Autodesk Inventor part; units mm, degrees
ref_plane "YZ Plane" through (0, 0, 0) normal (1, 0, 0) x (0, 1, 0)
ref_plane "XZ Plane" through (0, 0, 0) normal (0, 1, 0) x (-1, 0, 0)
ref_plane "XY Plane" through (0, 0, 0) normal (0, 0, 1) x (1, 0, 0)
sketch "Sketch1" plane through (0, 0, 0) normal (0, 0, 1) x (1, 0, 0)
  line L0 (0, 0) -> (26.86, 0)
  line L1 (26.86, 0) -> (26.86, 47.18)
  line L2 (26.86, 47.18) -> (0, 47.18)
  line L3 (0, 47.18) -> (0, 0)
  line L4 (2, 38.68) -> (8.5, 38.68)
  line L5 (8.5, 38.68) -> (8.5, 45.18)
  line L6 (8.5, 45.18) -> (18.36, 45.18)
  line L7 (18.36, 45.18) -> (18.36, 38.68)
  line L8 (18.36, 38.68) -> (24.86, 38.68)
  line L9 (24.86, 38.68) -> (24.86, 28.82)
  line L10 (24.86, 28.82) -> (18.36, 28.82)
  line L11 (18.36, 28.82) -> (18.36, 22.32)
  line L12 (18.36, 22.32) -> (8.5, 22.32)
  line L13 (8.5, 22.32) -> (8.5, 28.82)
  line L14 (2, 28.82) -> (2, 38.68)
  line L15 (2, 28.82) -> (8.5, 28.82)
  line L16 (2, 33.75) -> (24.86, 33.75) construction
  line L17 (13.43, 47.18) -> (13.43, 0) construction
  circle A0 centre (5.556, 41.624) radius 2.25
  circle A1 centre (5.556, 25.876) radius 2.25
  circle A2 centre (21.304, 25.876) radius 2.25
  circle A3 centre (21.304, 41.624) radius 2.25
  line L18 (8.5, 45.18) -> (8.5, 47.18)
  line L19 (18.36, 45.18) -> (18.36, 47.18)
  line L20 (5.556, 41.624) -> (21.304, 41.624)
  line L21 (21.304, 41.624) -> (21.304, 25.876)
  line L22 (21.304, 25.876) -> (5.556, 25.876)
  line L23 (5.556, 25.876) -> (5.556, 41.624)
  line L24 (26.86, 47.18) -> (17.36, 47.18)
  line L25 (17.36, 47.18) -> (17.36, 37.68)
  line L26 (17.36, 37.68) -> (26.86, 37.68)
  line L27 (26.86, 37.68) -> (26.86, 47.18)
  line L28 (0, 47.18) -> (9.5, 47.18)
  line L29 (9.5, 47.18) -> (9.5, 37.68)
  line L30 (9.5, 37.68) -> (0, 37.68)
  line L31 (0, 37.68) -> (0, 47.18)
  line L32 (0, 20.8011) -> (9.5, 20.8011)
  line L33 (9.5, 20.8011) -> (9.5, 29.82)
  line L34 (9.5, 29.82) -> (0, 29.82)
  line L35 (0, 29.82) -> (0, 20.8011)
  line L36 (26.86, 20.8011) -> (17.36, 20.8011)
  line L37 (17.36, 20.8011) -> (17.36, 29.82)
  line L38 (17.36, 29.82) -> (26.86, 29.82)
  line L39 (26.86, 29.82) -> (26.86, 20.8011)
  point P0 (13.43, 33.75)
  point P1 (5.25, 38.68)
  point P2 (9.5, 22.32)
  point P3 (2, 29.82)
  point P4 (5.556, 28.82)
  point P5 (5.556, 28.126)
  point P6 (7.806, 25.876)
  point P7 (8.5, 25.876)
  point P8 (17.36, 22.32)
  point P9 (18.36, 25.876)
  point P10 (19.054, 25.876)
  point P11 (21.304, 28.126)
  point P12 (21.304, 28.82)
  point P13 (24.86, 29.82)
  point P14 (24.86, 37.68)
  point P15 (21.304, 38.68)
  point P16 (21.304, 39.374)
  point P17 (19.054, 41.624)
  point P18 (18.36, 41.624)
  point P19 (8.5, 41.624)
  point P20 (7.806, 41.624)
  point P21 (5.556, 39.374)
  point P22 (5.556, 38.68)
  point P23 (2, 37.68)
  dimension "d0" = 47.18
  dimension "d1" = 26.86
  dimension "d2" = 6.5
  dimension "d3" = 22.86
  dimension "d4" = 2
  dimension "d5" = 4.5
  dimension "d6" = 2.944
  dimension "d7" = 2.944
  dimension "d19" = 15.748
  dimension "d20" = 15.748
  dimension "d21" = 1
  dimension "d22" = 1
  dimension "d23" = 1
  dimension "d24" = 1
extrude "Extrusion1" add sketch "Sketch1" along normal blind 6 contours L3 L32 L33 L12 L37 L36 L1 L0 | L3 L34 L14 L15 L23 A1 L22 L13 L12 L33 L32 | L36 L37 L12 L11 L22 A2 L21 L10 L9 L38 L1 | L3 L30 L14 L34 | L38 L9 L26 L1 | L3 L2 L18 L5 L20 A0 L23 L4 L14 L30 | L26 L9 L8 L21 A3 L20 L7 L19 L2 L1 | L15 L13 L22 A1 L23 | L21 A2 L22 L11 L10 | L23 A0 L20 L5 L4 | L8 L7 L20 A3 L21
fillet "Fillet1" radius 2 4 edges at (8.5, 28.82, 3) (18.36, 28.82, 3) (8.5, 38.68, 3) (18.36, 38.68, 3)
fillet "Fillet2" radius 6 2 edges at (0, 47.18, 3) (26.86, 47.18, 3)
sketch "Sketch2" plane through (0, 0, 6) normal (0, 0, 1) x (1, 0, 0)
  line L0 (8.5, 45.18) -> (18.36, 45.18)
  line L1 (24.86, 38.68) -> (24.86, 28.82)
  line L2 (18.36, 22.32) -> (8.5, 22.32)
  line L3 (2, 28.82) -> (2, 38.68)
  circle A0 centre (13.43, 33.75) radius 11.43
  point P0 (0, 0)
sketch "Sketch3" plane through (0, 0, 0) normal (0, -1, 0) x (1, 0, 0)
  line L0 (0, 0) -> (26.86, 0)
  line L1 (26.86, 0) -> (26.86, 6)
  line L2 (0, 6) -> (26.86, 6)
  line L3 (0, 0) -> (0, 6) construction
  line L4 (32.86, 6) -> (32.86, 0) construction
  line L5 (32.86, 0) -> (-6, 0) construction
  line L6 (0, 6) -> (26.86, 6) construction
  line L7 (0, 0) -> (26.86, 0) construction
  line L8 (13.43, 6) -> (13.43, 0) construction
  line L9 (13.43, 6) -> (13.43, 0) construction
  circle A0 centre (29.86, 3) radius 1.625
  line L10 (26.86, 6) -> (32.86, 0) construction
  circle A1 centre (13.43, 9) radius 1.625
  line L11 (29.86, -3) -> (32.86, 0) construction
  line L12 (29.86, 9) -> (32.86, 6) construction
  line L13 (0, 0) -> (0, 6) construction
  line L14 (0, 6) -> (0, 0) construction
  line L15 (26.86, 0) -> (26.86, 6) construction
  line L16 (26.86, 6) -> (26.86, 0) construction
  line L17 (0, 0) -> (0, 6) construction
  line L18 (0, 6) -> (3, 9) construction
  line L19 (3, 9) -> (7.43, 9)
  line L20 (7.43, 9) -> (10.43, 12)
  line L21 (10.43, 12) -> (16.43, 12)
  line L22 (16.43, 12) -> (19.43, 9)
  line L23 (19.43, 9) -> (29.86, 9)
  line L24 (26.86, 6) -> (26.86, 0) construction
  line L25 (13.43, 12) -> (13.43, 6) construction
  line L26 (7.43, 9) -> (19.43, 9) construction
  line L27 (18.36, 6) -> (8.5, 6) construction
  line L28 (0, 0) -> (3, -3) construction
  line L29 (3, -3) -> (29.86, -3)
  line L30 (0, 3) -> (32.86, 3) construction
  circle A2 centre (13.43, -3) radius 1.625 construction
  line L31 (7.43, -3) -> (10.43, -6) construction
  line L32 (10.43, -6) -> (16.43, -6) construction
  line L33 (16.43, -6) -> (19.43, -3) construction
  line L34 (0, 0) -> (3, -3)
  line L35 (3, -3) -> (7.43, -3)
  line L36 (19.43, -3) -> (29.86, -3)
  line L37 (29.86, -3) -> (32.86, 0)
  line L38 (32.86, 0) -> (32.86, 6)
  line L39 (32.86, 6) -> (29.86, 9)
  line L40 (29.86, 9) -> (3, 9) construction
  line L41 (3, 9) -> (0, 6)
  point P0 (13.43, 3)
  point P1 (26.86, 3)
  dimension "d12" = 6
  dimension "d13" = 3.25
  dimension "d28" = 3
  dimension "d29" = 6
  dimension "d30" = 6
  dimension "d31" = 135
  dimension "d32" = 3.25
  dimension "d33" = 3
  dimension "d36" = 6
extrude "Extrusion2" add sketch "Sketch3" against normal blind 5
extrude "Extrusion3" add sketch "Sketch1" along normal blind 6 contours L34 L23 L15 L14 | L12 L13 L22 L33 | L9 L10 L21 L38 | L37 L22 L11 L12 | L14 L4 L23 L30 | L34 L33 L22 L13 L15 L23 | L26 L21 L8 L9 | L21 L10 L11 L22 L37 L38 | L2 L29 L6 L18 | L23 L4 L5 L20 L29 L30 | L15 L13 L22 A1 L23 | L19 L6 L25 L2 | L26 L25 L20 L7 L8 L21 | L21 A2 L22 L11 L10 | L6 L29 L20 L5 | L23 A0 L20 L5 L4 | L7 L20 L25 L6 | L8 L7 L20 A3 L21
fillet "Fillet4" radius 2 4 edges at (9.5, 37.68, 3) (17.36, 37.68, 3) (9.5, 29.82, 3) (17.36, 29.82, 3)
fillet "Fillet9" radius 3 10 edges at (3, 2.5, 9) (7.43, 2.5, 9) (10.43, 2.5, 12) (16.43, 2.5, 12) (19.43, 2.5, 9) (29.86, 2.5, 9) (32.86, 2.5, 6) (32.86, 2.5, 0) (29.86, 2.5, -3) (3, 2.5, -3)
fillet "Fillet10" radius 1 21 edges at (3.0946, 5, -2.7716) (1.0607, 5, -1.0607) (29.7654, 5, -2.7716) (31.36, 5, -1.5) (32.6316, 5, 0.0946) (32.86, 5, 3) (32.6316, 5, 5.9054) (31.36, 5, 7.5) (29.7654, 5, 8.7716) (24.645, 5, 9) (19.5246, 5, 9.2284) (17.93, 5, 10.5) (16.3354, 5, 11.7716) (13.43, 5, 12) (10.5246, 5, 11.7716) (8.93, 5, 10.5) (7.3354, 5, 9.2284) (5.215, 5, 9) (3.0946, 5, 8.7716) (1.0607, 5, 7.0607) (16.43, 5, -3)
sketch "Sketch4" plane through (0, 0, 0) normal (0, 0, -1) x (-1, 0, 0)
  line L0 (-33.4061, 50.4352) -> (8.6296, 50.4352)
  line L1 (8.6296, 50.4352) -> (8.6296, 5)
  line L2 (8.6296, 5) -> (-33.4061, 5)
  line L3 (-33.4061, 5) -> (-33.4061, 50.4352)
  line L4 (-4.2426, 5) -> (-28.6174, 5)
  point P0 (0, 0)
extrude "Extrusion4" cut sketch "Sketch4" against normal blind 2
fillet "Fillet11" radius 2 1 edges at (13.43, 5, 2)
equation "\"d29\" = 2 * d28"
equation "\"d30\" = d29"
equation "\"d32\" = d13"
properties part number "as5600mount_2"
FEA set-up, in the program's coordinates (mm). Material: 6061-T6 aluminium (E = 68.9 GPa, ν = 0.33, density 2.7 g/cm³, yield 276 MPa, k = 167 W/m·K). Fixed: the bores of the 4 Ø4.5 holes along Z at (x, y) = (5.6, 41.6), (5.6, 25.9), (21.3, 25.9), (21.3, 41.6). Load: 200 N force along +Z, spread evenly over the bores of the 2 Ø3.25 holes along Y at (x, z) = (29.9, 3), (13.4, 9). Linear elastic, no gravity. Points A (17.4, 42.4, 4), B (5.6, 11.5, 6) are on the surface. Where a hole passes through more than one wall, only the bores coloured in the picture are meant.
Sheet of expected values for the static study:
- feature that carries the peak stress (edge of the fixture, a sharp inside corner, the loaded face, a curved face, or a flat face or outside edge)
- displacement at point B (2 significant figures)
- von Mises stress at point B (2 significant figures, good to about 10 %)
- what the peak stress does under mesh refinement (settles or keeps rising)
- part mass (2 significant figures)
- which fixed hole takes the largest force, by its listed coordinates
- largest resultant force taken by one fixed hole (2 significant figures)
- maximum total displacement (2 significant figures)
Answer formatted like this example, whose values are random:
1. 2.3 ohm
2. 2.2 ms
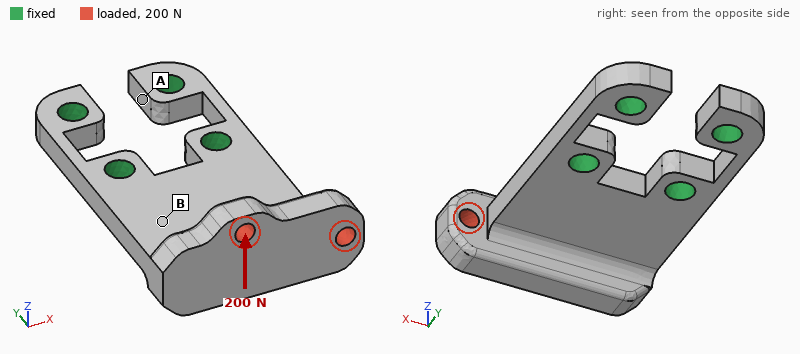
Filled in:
1. edge of the fixture
2. 0.033 mm
3. 28 MPa
4. keeps rising
5. 13 g
6. (21.3, 25.9)
7. 190 N
8. 0.13 mm
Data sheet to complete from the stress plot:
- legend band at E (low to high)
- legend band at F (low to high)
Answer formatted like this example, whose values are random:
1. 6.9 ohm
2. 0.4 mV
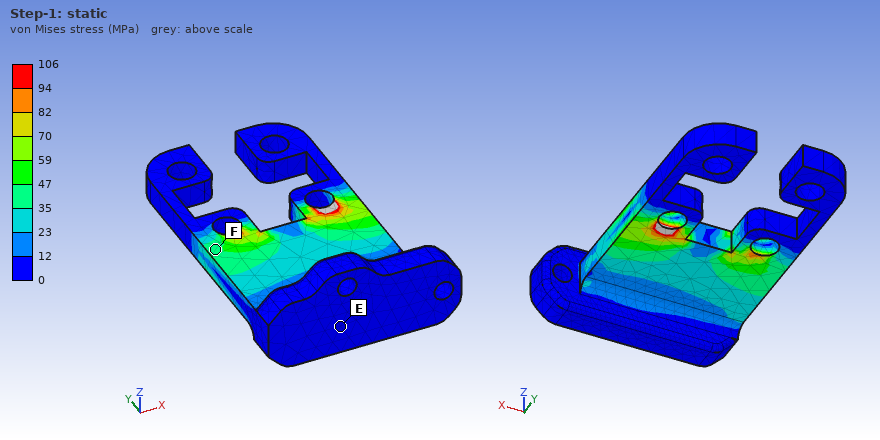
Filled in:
1. 0 to 12 MPa
2. 35 to 47 MPa
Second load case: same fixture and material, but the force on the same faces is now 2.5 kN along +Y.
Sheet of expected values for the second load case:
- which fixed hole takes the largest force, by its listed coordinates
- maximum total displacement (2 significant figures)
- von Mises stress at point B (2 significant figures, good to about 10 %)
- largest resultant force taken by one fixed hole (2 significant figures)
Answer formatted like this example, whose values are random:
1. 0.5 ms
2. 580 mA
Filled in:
1. (21.3, 25.9)
2. 0.20 mm
3. 69 MPa
4. 2.3 kN
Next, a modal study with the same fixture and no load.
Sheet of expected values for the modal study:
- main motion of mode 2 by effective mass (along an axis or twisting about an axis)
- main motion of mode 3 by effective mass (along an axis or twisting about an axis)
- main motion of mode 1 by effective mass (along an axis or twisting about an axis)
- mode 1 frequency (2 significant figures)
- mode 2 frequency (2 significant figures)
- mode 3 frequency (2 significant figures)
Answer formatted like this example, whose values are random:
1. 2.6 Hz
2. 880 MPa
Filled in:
1. twisting about Y
2. along X
3. along Z
4. 3000 Hz
5. 7300 Hz
6. 13 kHz
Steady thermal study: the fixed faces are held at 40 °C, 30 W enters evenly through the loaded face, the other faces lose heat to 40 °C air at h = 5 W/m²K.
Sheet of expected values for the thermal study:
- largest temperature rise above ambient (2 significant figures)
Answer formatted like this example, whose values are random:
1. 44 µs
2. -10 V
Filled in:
1. 56 K
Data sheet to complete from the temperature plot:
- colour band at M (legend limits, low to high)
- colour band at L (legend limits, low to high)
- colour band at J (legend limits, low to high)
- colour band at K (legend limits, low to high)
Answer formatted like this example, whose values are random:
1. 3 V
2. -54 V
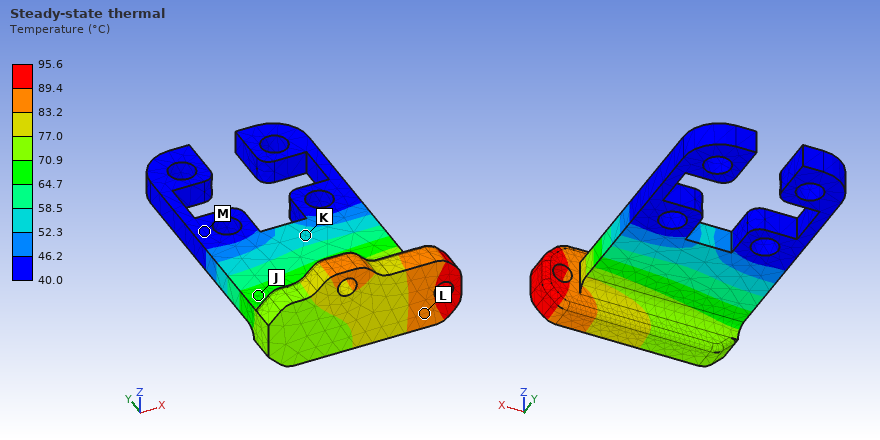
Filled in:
1. 40.0 to 46.2 °C
2. 83.2 to 89.4 °C
3. 64.7 to 70.9 °C
4. 52.3 to 58.5 °C
